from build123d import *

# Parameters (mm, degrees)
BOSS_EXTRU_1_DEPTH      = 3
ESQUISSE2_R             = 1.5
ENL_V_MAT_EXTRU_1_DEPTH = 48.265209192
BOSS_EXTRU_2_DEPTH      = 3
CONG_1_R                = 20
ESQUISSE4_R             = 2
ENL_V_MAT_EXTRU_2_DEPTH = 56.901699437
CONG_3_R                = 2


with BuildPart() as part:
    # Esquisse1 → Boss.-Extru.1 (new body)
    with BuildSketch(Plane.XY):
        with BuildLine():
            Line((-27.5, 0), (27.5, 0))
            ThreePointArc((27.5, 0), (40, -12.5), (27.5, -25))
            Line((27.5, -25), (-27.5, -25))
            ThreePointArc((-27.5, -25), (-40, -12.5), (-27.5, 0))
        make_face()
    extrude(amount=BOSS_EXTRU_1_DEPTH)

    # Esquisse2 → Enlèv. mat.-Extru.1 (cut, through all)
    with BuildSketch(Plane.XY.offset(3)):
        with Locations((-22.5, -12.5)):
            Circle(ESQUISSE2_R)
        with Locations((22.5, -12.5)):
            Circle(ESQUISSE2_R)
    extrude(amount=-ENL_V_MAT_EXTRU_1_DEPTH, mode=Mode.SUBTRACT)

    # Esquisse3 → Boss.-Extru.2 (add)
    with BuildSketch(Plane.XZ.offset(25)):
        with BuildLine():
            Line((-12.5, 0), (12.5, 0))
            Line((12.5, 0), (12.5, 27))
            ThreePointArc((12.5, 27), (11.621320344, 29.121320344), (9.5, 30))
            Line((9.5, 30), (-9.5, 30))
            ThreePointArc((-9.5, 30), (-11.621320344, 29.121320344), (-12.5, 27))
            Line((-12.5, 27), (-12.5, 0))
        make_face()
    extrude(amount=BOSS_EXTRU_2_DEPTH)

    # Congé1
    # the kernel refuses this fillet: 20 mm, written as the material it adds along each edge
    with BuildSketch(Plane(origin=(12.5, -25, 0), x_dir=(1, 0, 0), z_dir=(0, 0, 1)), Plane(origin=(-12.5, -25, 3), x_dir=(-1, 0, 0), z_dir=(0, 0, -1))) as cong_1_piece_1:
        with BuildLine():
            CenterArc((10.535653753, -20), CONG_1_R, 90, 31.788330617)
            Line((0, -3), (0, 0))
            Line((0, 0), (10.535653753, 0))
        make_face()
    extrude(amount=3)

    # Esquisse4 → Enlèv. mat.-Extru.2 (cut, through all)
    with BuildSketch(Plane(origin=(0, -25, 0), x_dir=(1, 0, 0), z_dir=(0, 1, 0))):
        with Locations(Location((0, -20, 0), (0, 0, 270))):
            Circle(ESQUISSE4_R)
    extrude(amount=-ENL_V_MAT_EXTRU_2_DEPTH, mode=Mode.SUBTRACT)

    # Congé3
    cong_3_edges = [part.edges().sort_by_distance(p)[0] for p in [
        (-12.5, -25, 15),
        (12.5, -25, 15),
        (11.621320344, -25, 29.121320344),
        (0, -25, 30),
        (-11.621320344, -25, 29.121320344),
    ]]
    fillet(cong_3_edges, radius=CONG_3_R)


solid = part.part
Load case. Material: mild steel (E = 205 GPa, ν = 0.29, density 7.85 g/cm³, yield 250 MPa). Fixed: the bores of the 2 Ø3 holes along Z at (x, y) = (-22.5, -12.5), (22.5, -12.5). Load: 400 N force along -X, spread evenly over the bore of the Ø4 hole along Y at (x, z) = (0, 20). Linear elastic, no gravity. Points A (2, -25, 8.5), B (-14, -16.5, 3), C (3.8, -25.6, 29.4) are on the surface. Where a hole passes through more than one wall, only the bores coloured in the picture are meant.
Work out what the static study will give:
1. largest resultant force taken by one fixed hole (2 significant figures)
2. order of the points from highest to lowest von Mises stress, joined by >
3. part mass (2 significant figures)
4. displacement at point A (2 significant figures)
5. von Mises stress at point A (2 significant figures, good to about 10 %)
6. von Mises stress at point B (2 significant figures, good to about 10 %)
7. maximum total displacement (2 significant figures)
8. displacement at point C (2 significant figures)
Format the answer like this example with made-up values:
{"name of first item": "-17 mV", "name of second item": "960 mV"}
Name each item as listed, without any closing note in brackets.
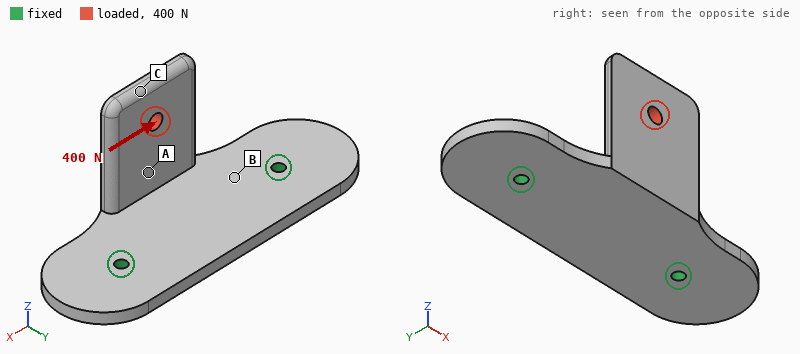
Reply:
{"largest resultant force taken by one fixed hole": "310 N", "order of the points from highest to lowest von Mises stress, joined by >": "B > A > C", "part mass": "61 g", "displacement at point A": "13 µm", "von Mises stress at point A": "23 MPa", "von Mises stress at point B": "40 MPa", "maximum total displacement": "51 µm", "displacement at point C": "48 µm"}
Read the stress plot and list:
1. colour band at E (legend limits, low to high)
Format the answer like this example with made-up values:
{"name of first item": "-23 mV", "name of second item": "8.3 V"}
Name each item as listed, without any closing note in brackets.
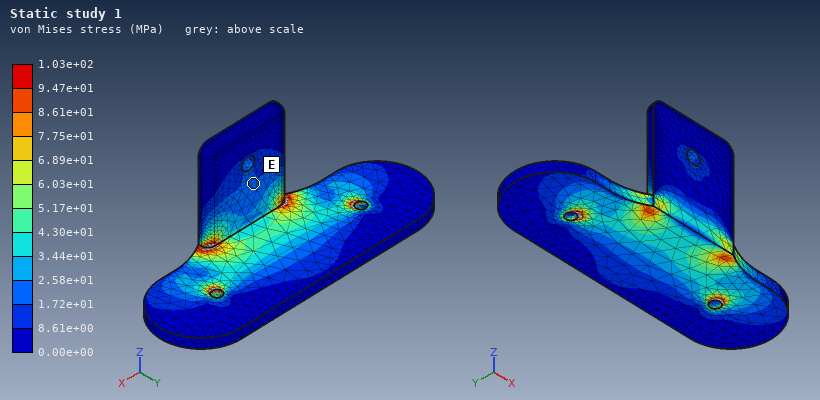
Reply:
{"colour band at E": "1.72e+01 to 2.58e+01 MPa"}
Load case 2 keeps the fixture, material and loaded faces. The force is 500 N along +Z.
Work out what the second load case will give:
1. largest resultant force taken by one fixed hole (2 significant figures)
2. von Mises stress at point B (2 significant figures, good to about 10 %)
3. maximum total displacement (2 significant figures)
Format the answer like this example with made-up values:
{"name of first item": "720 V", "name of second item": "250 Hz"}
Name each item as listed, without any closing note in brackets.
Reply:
{"largest resultant force taken by one fixed hole": "250 N", "von Mises stress at point B": "60 MPa", "maximum total displacement": "0.10 mm"}
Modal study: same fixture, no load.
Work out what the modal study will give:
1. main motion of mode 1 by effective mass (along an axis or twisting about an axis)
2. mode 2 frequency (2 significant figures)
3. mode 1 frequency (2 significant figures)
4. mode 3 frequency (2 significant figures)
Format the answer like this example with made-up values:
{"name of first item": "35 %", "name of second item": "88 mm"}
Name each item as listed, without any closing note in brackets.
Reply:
{"main motion of mode 1 by effective mass": "along Y", "mode 2 frequency": "4500 Hz", "mode 1 frequency": "2000 Hz", "mode 3 frequency": "4500 Hz"}
